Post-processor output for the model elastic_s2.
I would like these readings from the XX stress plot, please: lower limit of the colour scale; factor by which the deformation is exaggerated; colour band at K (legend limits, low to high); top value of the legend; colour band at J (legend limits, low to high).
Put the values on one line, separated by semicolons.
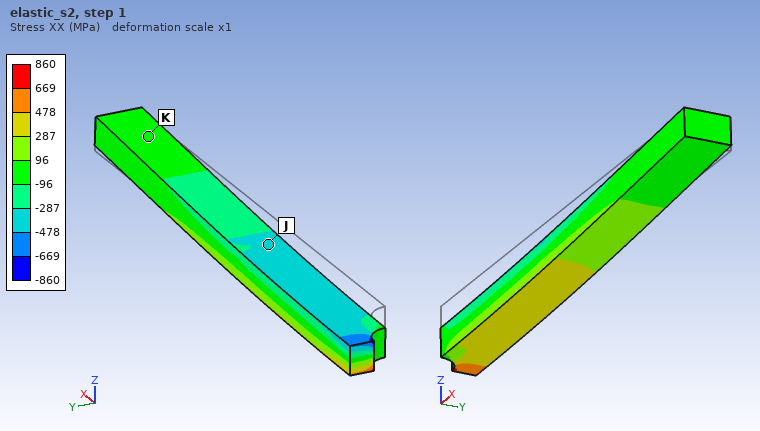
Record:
-860 MPa; 1; -96 to 96 MPa; 860 MPa; -478 to -287 MPa
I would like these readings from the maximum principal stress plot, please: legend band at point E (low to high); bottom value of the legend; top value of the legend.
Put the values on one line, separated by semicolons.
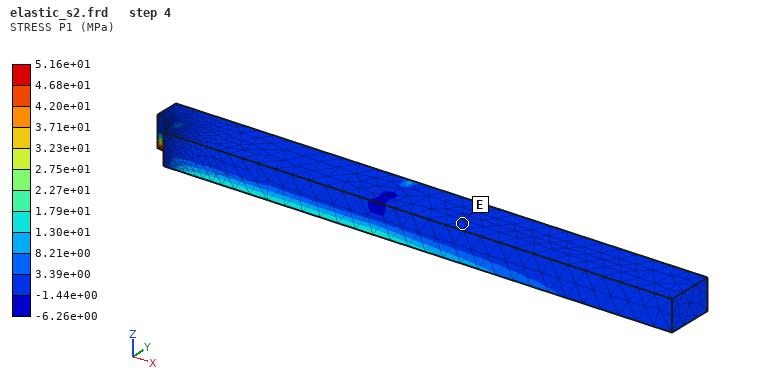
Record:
-1.44e+00 to 3.39e+00 MPa; -6.26e+00 MPa; 5.16e+01 MPa
